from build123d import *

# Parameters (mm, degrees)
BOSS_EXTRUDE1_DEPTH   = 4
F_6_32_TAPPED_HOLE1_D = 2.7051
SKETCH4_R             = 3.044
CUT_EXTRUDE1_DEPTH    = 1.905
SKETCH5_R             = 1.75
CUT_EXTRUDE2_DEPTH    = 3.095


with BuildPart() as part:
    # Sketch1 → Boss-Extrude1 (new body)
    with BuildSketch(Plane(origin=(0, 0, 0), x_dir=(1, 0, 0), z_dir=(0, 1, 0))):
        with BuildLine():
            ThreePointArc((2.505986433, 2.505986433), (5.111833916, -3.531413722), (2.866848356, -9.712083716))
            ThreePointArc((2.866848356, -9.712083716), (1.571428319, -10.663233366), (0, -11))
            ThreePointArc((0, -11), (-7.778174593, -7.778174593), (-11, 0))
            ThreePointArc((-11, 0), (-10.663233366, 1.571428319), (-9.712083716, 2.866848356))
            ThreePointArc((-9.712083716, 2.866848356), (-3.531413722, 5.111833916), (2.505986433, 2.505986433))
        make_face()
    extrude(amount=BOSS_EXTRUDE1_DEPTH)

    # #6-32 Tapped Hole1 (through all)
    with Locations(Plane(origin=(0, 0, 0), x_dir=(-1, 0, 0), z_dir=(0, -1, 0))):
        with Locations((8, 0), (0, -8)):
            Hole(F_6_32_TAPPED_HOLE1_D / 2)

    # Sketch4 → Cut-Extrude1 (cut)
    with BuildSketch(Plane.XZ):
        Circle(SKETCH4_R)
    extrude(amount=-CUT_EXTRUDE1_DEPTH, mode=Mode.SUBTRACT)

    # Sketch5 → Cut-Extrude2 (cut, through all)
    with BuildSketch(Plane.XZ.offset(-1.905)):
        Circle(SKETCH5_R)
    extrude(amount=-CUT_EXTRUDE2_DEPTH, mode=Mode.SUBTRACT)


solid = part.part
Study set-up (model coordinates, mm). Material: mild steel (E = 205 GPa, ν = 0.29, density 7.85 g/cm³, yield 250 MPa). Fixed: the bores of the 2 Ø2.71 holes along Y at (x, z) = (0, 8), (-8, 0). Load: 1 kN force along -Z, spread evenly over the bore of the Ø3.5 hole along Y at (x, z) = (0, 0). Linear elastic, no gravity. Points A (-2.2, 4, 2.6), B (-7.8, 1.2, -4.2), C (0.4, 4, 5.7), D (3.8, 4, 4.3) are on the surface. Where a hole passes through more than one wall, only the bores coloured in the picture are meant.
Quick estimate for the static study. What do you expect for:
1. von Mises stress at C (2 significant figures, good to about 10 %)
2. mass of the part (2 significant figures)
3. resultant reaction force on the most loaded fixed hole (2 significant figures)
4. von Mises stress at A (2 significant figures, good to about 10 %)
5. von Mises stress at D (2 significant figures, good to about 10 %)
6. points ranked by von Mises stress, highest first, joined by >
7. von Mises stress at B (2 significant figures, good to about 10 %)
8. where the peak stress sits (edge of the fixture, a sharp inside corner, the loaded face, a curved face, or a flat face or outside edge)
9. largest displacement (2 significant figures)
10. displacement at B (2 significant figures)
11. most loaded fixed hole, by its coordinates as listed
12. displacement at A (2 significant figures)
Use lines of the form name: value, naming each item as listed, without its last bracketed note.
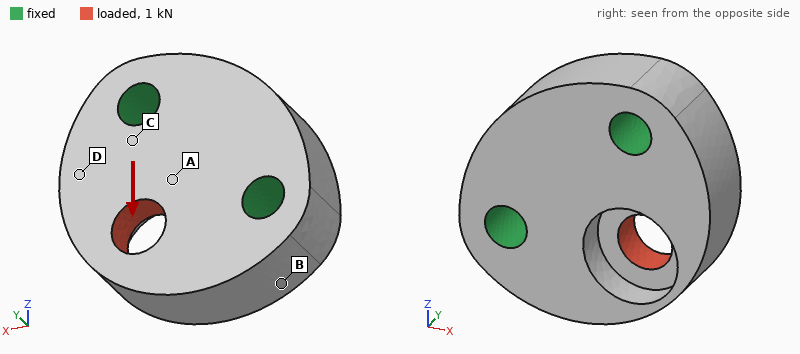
von Mises stress at C: 63 MPa
mass of the part: 5.3 g
resultant reaction force on the most loaded fixed hole: 770 N
von Mises stress at A: 47 MPa
von Mises stress at D: 34 MPa
points ranked by von Mises stress, highest first, joined by >: C > A > D > B
von Mises stress at B: 18 MPa
where the peak stress sits: the loaded face
largest displacement: 3.3 µm
displacement at B: 0.65 µm
most loaded fixed hole, by its coordinates as listed: (0, 8)
displacement at A: 0.93 µm
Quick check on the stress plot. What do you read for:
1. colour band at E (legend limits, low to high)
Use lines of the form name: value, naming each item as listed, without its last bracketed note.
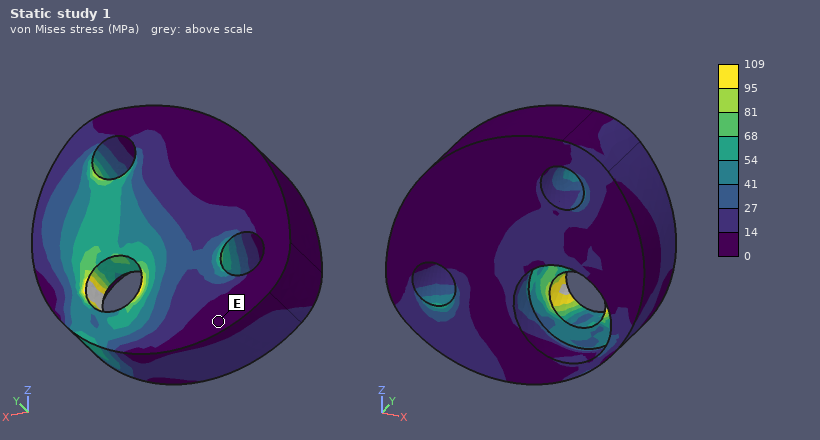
colour band at E: 0 to 14 MPa
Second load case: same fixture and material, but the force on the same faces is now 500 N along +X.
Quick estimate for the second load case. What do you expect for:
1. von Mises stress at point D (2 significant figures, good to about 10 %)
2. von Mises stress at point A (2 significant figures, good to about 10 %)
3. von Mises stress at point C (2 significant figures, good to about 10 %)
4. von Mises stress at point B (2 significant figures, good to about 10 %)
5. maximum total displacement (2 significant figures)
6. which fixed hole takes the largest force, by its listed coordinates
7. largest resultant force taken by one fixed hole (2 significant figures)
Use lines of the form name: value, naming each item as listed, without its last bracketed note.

von Mises stress at point D: 6.7 MPa
von Mises stress at point A: 23 MPa
von Mises stress at point C: 16 MPa
von Mises stress at point B: 6.8 MPa
maximum total displacement: 1.7 µm
which fixed hole takes the largest force, by its listed coordinates: (-8, 0)
largest resultant force taken by one fixed hole: 380 N
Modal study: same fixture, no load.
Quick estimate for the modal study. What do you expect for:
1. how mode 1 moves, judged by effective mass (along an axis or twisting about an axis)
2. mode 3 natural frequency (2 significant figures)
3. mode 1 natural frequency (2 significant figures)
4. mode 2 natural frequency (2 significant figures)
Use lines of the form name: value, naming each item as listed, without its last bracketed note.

how mode 1 moves, judged by effective mass: along Y
mode 3 natural frequency: 88 kHz
mode 1 natural frequency: 47 kHz
mode 2 natural frequency: 76 kHz
